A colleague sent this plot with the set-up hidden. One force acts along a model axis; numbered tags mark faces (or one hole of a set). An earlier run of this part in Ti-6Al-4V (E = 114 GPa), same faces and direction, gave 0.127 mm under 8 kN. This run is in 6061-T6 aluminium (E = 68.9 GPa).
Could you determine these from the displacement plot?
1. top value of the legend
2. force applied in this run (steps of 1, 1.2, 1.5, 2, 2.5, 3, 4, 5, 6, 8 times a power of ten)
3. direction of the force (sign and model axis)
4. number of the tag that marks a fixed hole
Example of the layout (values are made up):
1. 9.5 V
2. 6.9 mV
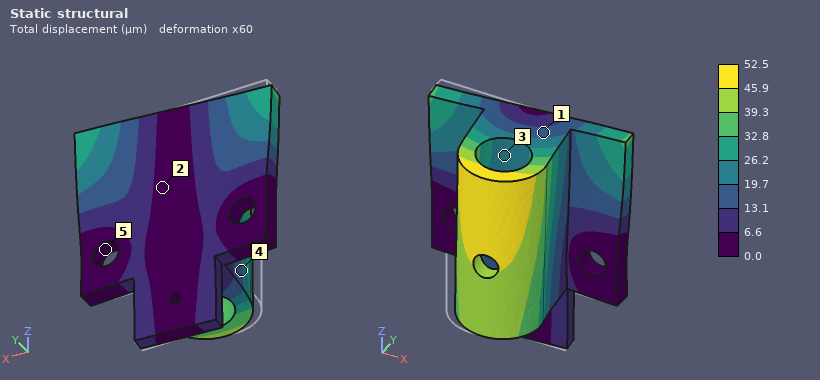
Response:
1. 52.5 µm
2. 2 kN
3. +X
4. 5
